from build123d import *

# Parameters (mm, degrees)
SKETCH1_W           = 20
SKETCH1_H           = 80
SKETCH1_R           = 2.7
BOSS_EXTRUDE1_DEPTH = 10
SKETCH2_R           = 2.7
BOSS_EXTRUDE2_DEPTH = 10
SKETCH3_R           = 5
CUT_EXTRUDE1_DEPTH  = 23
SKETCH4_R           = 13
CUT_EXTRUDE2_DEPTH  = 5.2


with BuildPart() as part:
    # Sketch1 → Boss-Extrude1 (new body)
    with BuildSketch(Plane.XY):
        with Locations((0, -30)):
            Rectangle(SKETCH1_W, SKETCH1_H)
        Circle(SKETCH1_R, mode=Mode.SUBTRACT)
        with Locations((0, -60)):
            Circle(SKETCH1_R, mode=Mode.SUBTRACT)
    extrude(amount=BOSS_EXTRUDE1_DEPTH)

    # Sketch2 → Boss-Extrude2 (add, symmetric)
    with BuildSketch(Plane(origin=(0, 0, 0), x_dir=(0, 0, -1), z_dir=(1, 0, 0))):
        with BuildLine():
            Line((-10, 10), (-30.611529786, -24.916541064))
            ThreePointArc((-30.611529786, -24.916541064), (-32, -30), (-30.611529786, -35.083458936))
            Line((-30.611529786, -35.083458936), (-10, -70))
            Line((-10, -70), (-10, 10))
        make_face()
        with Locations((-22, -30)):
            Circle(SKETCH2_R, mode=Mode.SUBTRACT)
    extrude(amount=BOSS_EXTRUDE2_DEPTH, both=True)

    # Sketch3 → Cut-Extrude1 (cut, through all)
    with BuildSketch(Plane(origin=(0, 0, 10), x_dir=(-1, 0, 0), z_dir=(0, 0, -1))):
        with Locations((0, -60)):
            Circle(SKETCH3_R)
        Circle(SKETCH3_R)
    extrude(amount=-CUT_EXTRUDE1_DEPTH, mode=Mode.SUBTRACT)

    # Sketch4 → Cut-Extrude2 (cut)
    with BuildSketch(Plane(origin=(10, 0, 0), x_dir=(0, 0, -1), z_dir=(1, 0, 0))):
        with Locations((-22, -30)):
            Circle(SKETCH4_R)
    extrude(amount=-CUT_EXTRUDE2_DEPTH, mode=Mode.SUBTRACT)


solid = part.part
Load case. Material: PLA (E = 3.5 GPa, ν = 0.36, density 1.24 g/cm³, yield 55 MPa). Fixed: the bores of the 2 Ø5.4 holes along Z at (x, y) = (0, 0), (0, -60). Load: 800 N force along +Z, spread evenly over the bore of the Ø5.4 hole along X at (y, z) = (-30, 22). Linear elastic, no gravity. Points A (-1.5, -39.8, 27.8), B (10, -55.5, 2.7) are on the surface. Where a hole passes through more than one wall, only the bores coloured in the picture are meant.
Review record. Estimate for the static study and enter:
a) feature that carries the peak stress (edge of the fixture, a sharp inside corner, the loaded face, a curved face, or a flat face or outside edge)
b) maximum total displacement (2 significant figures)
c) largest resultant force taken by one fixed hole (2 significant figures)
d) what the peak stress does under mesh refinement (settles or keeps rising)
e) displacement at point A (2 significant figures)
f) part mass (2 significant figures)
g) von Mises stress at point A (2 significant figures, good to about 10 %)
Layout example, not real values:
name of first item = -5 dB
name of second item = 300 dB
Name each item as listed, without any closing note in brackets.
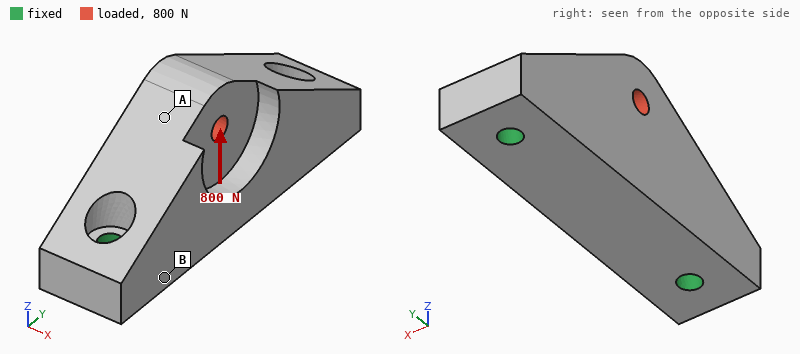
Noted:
feature that carries the peak stress = edge of the fixture
maximum total displacement = 69 µm
largest resultant force taken by one fixed hole = 480 N
what the peak stress does under mesh refinement = keeps rising
displacement at point A = 50 µm
part mass = 38 g
von Mises stress at point A = 3.4 MPa
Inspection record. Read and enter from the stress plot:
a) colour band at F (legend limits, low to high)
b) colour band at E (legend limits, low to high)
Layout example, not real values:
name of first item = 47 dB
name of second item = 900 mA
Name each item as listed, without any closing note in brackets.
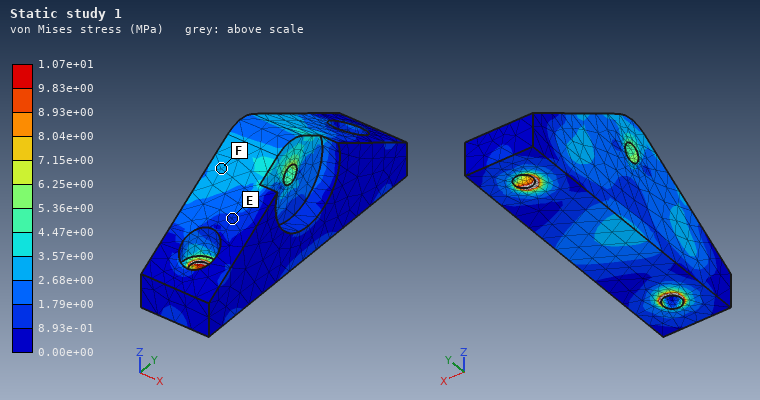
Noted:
colour band at F = 2.68e+00 to 3.57e+00 MPa
colour band at E = 8.93e-01 to 1.79e+00 MPa
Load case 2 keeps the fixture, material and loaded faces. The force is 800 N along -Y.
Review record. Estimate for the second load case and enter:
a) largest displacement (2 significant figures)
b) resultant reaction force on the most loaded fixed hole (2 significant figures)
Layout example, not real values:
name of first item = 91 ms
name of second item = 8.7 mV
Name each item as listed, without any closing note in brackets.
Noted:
largest displacement = 28 µm
resultant reaction force on the most loaded fixed hole = 460 N
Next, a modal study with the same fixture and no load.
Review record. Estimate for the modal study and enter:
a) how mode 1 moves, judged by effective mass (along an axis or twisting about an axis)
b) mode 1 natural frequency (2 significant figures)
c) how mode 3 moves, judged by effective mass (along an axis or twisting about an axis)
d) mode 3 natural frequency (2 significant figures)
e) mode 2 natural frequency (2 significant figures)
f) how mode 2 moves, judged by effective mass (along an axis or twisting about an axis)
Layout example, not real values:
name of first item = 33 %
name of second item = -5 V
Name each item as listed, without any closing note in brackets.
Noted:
how mode 1 moves, judged by effective mass = along X
mode 1 natural frequency = 2800 Hz
how mode 3 moves, judged by effective mass = along X
mode 3 natural frequency = 5300 Hz
mode 2 natural frequency = 4900 Hz
how mode 2 moves, judged by effective mass = along Z
